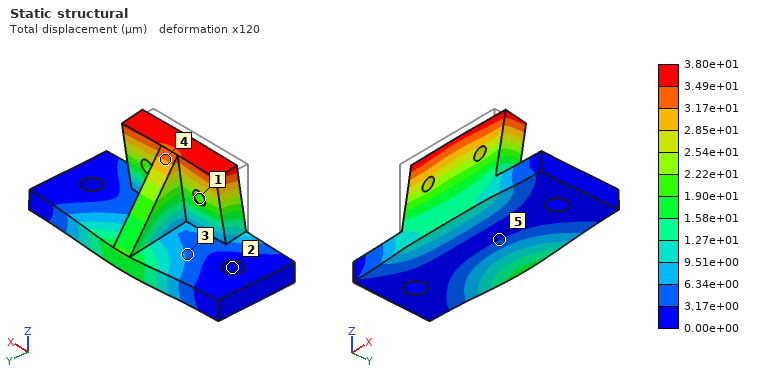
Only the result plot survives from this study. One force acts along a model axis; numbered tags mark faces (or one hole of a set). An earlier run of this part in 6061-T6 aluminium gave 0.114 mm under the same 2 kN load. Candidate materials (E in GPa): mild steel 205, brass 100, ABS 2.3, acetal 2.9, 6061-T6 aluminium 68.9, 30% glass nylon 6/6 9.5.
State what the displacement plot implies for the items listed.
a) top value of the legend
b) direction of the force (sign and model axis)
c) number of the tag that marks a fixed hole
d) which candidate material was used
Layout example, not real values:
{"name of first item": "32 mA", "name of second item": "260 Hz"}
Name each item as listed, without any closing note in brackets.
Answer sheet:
{"top value of the legend": "3.80e+01 µm", "direction of the force": "+Y", "number of the tag that marks a fixed hole": "2", "which candidate material was used": "mild steel"}
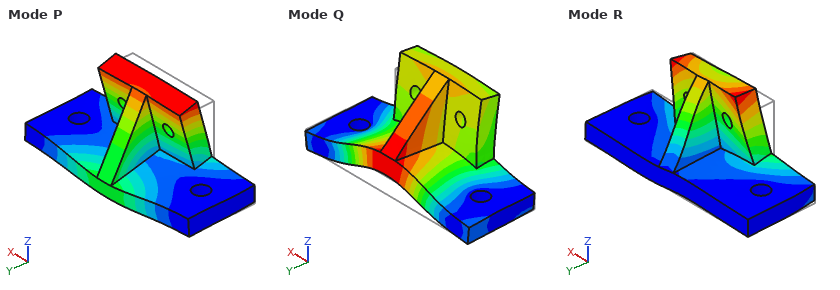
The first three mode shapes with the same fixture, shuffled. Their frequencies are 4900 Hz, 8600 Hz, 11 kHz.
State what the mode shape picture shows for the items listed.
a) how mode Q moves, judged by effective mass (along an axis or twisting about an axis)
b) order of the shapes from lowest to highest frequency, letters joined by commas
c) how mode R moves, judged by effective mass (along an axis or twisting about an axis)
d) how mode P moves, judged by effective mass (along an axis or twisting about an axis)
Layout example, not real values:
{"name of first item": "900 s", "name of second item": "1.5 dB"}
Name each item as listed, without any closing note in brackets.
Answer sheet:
{"how mode Q moves, judged by effective mass": "along Z", "order of the shapes from lowest to highest frequency, letters joined by commas": "P, Q, R", "how mode R moves, judged by effective mass": "along X", "how mode P moves, judged by effective mass": "along Y"}
